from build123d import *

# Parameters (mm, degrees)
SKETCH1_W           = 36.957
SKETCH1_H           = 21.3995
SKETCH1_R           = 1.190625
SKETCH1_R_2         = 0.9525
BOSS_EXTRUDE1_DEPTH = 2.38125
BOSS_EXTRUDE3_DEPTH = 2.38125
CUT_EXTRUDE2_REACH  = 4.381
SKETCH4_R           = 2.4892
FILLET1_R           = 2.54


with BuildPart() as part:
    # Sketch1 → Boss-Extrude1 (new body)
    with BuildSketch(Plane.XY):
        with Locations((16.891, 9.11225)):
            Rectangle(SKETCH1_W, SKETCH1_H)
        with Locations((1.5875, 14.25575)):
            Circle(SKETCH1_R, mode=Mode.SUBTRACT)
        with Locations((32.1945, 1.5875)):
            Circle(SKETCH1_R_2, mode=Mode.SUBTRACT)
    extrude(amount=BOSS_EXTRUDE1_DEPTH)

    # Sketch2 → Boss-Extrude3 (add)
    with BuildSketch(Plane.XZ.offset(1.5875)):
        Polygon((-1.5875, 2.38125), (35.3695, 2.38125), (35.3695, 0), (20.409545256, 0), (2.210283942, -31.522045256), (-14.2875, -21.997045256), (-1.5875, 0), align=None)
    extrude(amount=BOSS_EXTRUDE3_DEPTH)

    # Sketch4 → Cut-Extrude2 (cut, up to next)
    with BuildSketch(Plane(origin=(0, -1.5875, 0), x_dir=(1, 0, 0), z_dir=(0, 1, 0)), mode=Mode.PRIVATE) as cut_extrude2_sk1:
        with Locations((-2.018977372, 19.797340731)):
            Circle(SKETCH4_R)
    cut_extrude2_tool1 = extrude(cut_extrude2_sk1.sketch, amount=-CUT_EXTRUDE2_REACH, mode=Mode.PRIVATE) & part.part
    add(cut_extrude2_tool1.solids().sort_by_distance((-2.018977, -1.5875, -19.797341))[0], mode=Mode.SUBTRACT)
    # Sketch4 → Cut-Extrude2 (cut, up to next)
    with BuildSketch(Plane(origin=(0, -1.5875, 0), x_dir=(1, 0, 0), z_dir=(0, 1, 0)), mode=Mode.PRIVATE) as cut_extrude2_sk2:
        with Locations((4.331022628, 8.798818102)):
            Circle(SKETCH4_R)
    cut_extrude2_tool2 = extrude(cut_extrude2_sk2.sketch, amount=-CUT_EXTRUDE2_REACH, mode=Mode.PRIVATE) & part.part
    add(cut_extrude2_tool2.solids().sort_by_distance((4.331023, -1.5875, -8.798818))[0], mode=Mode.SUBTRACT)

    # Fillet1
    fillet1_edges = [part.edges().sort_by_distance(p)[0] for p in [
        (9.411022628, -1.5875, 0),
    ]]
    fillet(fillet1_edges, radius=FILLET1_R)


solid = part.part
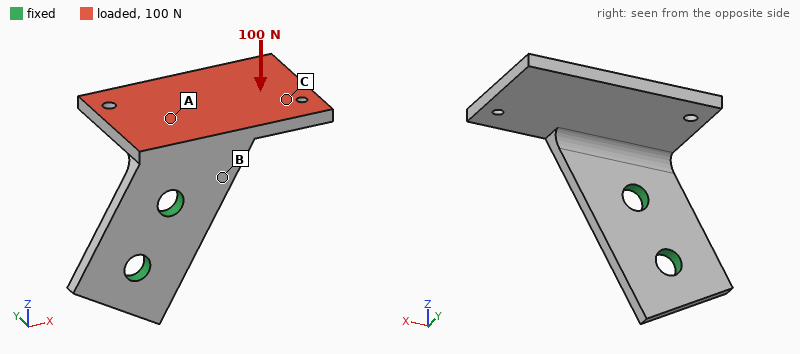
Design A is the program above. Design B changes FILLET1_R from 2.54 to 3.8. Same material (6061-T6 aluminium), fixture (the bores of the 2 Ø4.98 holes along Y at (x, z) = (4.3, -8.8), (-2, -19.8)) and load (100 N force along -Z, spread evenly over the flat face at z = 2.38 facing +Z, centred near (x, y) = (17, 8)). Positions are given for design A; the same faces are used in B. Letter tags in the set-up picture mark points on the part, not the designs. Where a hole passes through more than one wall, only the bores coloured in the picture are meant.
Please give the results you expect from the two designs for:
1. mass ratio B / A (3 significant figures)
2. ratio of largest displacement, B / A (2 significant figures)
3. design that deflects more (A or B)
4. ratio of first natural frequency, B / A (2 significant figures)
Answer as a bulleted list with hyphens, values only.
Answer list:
- 1.01
- 0.89
- A
- 1.1
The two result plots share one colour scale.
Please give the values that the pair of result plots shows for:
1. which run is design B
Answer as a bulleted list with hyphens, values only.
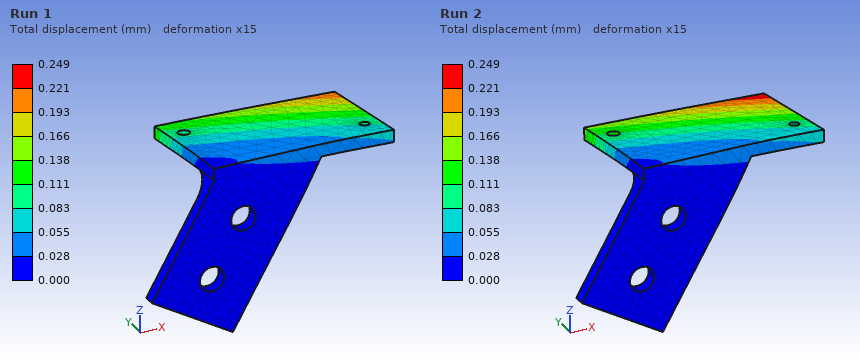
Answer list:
- Run 1
